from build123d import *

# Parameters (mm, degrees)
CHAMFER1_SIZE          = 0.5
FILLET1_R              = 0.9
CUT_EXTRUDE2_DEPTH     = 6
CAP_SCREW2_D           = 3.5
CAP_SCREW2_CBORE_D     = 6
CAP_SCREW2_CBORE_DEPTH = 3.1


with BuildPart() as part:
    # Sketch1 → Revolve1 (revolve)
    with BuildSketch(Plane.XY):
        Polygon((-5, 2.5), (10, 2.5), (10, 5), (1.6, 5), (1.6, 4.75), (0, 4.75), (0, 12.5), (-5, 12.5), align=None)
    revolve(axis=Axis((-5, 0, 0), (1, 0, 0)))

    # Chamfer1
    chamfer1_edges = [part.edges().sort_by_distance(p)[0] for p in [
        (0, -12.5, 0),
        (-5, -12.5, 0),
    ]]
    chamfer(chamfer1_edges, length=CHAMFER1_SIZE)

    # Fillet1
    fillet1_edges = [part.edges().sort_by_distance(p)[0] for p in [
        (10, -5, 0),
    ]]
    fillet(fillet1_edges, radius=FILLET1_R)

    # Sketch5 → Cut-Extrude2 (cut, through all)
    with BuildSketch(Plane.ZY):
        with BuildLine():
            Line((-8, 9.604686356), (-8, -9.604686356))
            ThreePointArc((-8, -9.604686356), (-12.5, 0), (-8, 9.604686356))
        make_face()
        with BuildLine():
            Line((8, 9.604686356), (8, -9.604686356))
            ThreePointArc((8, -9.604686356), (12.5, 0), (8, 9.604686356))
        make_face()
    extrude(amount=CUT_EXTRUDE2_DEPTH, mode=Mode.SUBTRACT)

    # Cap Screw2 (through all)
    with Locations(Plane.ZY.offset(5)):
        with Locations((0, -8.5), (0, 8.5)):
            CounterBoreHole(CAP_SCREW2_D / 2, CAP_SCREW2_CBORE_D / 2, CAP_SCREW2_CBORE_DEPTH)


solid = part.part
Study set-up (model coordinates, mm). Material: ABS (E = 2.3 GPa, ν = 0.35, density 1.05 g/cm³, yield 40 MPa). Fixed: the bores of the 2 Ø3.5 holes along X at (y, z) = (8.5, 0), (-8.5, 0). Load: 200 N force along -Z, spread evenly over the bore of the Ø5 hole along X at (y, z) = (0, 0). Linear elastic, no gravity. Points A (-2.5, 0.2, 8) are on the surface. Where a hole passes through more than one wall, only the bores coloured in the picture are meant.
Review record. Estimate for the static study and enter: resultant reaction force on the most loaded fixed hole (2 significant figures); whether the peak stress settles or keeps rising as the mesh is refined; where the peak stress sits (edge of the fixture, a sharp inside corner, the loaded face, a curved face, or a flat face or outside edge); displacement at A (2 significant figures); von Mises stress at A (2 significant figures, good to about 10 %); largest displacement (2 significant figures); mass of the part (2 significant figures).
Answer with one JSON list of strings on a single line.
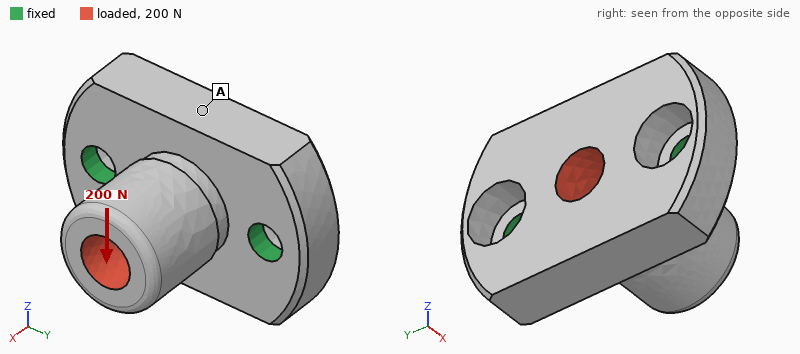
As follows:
["100 N", "keeps rising", "edge of the fixture", "0.11 mm", "3.8 MPa", "0.23 mm", "2.2 g"]
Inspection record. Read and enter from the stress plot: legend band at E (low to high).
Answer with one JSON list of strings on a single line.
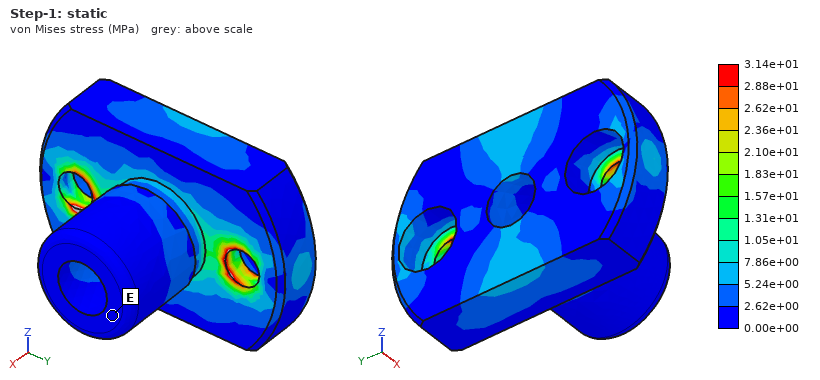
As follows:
["0.00e+00 to 2.62e+00 MPa"]
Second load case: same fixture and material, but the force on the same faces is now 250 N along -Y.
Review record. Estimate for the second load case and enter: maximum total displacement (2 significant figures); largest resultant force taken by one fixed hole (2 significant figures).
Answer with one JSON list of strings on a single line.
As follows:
["0.11 mm", "140 N"]
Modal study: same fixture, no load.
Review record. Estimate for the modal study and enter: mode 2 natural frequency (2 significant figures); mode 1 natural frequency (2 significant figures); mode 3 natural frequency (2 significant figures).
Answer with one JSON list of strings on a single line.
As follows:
["9100 Hz", "4200 Hz", "9200 Hz"]
